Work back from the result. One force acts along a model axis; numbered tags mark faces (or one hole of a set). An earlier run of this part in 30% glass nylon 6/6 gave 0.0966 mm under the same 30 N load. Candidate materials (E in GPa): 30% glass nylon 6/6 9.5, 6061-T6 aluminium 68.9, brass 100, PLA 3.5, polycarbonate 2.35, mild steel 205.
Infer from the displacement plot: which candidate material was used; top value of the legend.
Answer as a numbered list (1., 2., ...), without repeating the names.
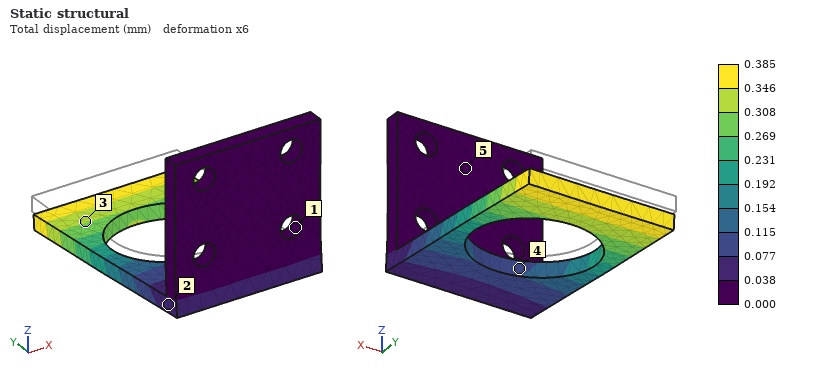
1. polycarbonate
2. 0.385 mm
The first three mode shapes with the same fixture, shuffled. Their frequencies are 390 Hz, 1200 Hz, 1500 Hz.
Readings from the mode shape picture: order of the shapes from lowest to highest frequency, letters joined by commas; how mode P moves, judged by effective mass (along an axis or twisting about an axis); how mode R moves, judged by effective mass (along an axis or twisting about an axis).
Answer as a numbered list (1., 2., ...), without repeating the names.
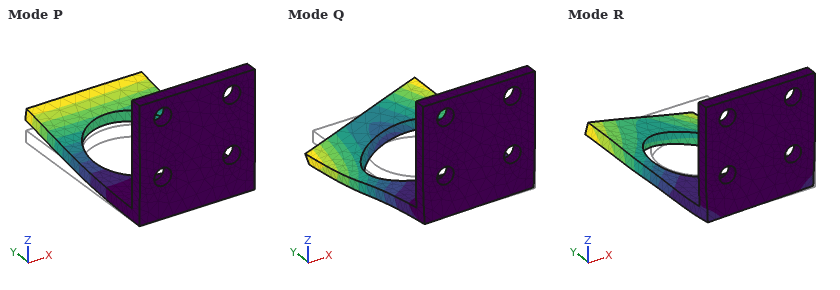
1. P, Q, R
2. along Z
3. along X
